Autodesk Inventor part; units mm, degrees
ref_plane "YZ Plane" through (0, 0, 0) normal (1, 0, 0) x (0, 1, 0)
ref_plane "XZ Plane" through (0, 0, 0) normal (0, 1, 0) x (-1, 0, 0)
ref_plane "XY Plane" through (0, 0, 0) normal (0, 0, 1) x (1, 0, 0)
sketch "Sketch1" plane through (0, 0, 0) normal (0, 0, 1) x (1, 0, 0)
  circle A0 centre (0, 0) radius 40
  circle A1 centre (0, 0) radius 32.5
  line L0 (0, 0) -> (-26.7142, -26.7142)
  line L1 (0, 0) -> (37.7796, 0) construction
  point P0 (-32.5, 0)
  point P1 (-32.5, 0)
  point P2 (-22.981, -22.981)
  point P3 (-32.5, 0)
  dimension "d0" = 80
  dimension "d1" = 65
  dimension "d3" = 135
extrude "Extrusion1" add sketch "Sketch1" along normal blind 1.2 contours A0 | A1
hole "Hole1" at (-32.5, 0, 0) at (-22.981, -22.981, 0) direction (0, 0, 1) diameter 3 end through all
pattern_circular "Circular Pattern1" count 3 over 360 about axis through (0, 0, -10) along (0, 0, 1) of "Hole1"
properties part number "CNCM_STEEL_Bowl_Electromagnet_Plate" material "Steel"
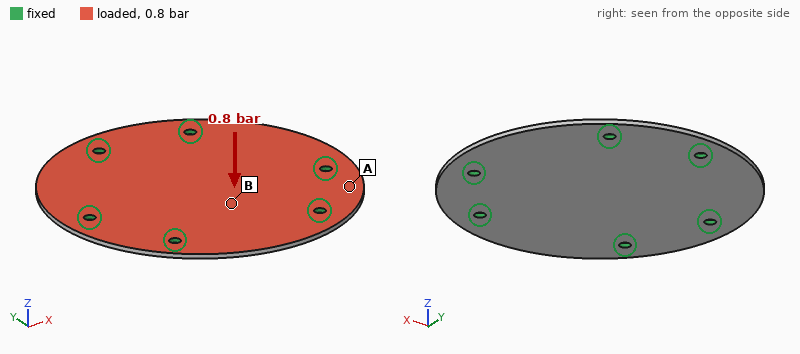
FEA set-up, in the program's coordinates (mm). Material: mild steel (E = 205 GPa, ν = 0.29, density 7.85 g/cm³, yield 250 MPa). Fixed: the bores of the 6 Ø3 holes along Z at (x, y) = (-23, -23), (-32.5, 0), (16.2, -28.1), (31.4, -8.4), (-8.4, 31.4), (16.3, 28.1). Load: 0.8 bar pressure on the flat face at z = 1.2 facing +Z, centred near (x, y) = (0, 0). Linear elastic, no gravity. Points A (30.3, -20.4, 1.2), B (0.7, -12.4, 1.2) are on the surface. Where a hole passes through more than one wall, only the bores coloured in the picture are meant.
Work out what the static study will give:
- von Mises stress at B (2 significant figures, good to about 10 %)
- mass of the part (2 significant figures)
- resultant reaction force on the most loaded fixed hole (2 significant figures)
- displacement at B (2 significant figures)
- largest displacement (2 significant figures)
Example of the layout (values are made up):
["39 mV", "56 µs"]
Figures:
["25 MPa", "47 g", "66 N", "42 µm", "53 µm"]
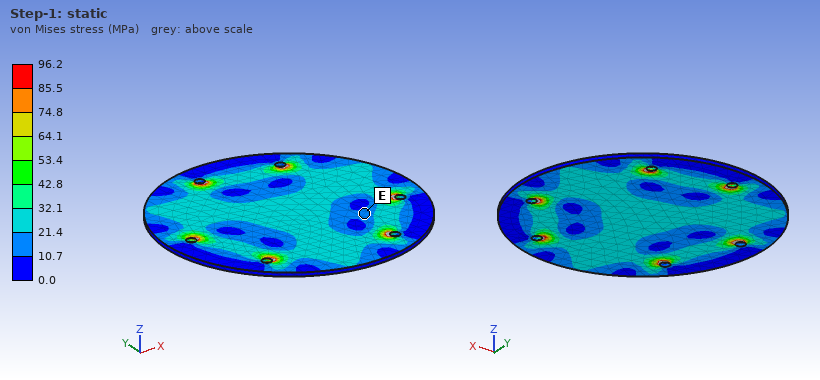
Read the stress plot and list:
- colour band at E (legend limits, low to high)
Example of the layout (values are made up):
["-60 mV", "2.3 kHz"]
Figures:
["10.7 to 21.4 MPa"]
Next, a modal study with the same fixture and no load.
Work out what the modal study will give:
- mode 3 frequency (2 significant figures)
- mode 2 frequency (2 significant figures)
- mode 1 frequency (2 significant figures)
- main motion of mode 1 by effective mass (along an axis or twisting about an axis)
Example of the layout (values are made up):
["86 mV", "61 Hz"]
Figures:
["3400 Hz", "3400 Hz", "2400 Hz", "along Z"]
